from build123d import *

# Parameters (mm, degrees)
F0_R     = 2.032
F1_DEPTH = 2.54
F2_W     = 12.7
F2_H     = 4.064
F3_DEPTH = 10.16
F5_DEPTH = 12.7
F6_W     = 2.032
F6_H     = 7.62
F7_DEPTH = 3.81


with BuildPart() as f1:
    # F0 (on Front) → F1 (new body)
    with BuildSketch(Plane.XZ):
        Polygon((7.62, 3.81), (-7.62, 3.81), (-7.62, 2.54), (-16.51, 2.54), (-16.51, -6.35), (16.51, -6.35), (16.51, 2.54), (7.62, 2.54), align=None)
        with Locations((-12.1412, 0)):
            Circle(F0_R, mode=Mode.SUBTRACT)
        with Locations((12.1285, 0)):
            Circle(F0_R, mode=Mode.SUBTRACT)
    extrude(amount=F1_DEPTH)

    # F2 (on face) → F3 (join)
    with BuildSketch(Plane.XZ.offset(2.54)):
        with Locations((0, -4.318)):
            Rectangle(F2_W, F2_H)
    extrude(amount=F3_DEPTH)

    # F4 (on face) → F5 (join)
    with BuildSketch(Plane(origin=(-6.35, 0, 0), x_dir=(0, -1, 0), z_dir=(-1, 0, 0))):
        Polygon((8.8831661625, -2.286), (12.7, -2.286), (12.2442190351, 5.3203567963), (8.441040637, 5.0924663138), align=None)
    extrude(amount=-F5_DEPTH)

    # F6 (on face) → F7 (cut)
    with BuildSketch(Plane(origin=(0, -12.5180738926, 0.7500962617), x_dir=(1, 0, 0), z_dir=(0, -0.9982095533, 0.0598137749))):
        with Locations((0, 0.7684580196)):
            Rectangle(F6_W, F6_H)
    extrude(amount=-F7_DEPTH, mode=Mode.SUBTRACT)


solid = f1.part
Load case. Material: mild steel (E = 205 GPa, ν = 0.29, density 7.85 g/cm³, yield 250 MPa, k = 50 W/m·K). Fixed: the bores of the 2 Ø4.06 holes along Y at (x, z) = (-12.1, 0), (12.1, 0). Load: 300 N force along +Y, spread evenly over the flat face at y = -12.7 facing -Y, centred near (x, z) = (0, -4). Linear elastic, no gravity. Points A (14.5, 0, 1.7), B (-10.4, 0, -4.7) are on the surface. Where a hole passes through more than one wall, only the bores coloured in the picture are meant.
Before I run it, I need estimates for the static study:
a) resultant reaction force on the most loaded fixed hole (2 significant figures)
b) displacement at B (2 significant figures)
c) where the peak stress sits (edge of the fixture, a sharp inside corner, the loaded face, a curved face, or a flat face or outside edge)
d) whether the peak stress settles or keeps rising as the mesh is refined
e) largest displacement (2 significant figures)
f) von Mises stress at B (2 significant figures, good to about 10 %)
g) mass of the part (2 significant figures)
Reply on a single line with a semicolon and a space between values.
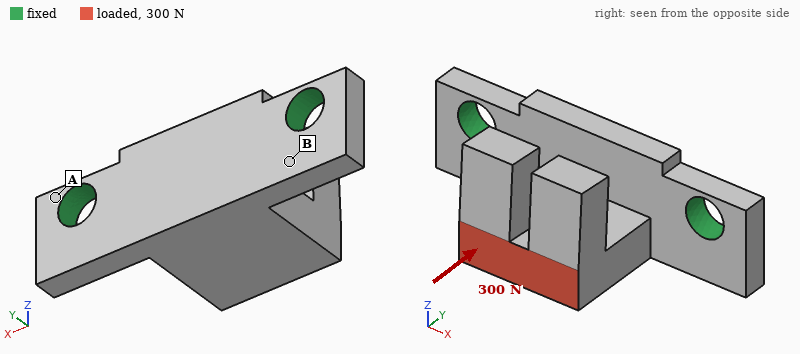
160 N; 1.6 µm; edge of the fixture; keeps rising; 9.7 µm; 35 MPa; 12 g
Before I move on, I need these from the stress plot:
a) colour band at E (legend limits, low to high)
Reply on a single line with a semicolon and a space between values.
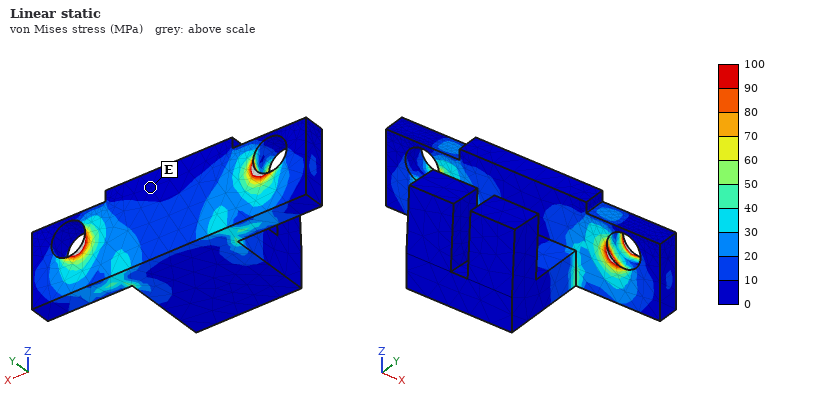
0 to 10 MPa
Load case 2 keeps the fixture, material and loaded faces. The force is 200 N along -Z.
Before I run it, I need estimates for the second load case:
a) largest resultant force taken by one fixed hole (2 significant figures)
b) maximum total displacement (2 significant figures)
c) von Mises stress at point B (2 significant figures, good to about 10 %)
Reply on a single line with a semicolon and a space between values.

100 N; 37 µm; 67 MPa
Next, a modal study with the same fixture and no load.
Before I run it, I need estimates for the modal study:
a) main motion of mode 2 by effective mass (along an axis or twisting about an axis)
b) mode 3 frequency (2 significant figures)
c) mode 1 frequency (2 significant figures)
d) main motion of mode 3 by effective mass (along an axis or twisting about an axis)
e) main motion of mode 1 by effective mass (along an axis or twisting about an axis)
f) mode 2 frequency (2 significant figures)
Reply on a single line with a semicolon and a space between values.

along X; 16 kHz; 6700 Hz; along Y; along Z; 14 kHz
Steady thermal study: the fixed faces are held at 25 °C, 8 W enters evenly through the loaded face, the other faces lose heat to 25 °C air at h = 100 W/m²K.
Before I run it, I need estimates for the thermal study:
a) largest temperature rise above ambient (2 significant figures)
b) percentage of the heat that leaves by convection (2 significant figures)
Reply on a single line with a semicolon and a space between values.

45 K; 33 %
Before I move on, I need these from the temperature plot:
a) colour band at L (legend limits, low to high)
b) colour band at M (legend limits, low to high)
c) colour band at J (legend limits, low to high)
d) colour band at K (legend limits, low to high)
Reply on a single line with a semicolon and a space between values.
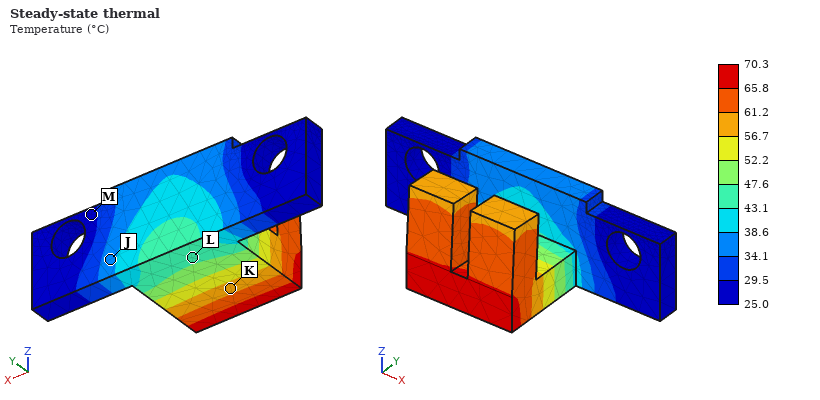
43.1 to 47.6 °C; 25.0 to 29.5 °C; 34.1 to 38.6 °C; 56.7 to 61.2 °C
